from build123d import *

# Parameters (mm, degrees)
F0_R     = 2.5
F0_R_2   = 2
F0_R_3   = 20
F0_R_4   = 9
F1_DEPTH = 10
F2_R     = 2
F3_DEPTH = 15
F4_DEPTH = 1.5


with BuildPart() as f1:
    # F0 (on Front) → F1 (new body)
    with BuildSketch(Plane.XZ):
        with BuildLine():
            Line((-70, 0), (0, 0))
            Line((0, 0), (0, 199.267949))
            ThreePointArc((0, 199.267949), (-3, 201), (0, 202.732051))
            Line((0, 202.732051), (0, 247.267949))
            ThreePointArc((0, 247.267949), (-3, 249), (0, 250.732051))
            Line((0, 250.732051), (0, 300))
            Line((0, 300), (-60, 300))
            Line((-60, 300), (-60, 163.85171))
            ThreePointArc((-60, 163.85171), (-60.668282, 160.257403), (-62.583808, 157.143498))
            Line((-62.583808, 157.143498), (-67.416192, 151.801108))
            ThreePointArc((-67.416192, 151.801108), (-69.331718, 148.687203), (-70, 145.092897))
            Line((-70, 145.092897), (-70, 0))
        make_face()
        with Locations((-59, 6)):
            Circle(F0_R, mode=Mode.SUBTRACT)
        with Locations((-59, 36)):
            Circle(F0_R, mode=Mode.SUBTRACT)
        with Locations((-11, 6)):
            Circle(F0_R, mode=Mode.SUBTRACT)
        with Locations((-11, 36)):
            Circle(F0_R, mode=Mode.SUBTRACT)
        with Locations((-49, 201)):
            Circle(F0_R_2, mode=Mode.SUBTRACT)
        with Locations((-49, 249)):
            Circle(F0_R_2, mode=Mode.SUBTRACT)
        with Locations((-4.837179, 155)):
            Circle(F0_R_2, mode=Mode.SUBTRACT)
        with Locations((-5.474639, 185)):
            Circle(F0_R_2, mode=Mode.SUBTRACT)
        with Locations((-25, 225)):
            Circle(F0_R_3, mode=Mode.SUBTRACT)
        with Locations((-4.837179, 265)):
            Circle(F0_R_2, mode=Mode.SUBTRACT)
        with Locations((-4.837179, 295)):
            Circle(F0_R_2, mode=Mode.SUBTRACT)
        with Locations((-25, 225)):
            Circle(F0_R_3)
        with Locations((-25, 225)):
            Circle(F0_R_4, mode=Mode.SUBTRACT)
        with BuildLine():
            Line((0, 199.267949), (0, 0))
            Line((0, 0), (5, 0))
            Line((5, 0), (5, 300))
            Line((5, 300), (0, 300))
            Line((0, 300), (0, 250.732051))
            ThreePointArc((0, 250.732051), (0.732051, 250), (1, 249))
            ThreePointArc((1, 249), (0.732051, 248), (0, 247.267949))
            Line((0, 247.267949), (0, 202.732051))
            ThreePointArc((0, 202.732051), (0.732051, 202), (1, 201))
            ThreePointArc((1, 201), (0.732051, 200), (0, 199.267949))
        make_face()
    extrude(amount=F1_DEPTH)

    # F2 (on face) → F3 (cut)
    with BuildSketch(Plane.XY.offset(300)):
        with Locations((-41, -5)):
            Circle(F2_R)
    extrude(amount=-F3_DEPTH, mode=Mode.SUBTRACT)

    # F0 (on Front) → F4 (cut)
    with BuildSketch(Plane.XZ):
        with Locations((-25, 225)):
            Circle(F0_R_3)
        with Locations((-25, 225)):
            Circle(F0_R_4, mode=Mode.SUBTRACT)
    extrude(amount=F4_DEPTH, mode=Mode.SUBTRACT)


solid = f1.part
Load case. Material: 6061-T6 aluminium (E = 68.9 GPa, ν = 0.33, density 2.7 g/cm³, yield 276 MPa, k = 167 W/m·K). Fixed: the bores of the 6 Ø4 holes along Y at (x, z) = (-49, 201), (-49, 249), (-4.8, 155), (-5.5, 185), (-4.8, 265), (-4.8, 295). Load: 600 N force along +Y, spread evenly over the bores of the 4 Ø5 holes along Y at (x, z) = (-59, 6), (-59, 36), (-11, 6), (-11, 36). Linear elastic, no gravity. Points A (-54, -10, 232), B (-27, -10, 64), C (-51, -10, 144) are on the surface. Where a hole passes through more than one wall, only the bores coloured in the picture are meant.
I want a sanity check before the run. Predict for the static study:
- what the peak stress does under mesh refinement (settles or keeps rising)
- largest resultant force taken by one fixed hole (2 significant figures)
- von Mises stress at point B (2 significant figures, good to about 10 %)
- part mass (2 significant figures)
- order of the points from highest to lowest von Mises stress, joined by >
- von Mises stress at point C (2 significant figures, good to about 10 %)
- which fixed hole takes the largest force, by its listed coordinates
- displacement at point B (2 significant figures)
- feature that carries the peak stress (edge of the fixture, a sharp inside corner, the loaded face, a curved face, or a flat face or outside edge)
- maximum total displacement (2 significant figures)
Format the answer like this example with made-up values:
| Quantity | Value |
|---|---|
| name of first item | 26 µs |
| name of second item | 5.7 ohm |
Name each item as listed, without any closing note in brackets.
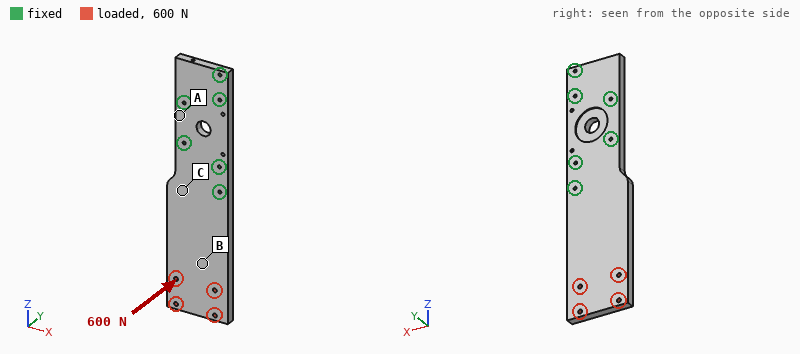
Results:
| Quantity | Value |
|---|---|
| what the peak stress does under mesh refinement | keeps rising |
| largest resultant force taken by one fixed hole | 1.9 kN |
| von Mises stress at point B | 20 MPa |
| part mass | 550 g |
| order of the points from highest to lowest von Mises stress, joined by > | C > B > A |
| von Mises stress at point C | 47 MPa |
| which fixed hole takes the largest force, by its listed coordinates | (-4.8, 155) |
| displacement at point B | 0.85 mm |
| feature that carries the peak stress | edge of the fixture |
| maximum total displacement | 1.9 mm |
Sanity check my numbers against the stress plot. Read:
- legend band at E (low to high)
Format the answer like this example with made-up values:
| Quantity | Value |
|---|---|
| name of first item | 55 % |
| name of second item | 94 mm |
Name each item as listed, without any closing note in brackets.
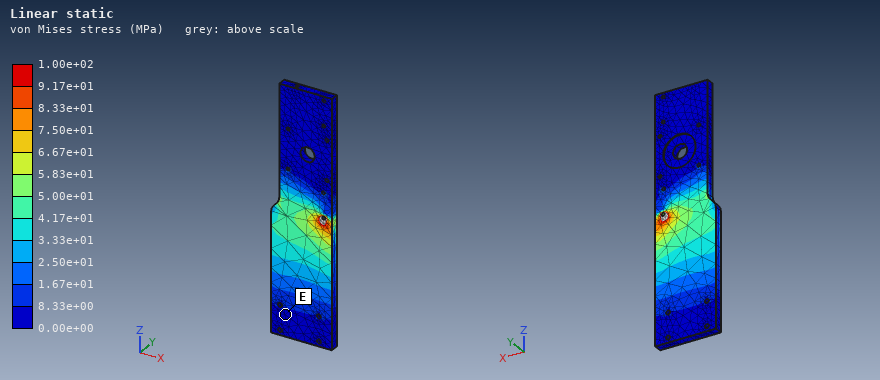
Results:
| Quantity | Value |
|---|---|
| legend band at E | 0.00e+00 to 8.33e+00 MPa |
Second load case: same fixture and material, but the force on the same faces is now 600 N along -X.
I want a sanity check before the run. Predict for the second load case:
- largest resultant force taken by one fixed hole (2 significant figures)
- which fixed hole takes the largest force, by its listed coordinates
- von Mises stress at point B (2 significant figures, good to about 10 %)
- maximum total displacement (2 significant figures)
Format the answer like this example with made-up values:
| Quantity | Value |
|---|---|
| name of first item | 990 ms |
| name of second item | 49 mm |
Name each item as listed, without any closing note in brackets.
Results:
| Quantity | Value |
|---|---|
| largest resultant force taken by one fixed hole | 1.8 kN |
| which fixed hole takes the largest force, by its listed coordinates | (-4.8, 155) |
| von Mises stress at point B | 2.1 MPa |
| maximum total displacement | 53 µm |
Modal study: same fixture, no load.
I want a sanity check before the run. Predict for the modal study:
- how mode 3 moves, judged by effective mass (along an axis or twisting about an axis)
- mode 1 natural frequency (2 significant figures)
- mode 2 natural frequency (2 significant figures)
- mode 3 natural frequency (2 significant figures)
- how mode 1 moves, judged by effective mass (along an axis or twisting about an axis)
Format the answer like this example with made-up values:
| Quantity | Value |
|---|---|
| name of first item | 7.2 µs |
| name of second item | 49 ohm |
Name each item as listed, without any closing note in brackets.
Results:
| Quantity | Value |
|---|---|
| how mode 3 moves, judged by effective mass | along X |
| mode 1 natural frequency | 290 Hz |
| mode 2 natural frequency | 1100 Hz |
| mode 3 natural frequency | 1600 Hz |
| how mode 1 moves, judged by effective mass | along Y |
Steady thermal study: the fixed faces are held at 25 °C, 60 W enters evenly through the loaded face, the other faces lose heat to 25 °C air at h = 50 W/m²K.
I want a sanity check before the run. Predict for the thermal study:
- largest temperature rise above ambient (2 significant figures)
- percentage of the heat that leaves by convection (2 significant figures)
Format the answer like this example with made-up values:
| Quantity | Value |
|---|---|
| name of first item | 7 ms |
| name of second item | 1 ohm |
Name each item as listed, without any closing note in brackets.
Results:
| Quantity | Value |
|---|---|
| largest temperature rise above ambient | 46 K |
| percentage of the heat that leaves by convection | 56 % |
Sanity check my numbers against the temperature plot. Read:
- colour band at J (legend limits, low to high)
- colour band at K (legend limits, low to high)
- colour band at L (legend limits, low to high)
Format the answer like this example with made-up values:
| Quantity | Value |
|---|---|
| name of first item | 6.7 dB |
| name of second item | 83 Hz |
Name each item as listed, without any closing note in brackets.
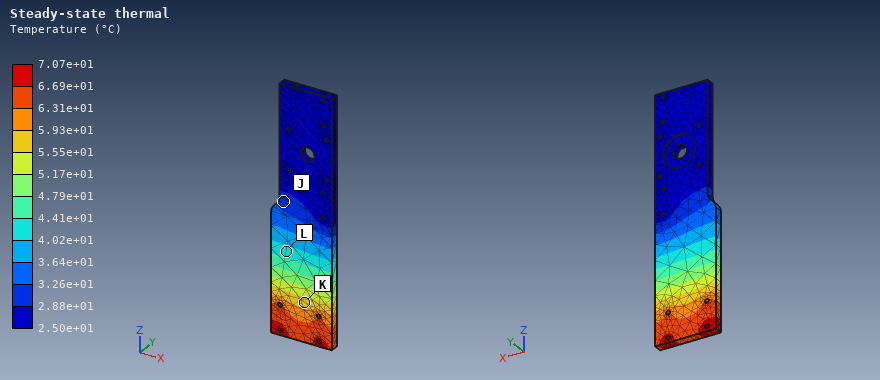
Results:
| Quantity | Value |
|---|---|
| colour band at J | 2.88e+01 to 3.26e+01 °C |
| colour band at K | 5.55e+01 to 5.93e+01 °C |
| colour band at L | 4.02e+01 to 4.41e+01 °C |
